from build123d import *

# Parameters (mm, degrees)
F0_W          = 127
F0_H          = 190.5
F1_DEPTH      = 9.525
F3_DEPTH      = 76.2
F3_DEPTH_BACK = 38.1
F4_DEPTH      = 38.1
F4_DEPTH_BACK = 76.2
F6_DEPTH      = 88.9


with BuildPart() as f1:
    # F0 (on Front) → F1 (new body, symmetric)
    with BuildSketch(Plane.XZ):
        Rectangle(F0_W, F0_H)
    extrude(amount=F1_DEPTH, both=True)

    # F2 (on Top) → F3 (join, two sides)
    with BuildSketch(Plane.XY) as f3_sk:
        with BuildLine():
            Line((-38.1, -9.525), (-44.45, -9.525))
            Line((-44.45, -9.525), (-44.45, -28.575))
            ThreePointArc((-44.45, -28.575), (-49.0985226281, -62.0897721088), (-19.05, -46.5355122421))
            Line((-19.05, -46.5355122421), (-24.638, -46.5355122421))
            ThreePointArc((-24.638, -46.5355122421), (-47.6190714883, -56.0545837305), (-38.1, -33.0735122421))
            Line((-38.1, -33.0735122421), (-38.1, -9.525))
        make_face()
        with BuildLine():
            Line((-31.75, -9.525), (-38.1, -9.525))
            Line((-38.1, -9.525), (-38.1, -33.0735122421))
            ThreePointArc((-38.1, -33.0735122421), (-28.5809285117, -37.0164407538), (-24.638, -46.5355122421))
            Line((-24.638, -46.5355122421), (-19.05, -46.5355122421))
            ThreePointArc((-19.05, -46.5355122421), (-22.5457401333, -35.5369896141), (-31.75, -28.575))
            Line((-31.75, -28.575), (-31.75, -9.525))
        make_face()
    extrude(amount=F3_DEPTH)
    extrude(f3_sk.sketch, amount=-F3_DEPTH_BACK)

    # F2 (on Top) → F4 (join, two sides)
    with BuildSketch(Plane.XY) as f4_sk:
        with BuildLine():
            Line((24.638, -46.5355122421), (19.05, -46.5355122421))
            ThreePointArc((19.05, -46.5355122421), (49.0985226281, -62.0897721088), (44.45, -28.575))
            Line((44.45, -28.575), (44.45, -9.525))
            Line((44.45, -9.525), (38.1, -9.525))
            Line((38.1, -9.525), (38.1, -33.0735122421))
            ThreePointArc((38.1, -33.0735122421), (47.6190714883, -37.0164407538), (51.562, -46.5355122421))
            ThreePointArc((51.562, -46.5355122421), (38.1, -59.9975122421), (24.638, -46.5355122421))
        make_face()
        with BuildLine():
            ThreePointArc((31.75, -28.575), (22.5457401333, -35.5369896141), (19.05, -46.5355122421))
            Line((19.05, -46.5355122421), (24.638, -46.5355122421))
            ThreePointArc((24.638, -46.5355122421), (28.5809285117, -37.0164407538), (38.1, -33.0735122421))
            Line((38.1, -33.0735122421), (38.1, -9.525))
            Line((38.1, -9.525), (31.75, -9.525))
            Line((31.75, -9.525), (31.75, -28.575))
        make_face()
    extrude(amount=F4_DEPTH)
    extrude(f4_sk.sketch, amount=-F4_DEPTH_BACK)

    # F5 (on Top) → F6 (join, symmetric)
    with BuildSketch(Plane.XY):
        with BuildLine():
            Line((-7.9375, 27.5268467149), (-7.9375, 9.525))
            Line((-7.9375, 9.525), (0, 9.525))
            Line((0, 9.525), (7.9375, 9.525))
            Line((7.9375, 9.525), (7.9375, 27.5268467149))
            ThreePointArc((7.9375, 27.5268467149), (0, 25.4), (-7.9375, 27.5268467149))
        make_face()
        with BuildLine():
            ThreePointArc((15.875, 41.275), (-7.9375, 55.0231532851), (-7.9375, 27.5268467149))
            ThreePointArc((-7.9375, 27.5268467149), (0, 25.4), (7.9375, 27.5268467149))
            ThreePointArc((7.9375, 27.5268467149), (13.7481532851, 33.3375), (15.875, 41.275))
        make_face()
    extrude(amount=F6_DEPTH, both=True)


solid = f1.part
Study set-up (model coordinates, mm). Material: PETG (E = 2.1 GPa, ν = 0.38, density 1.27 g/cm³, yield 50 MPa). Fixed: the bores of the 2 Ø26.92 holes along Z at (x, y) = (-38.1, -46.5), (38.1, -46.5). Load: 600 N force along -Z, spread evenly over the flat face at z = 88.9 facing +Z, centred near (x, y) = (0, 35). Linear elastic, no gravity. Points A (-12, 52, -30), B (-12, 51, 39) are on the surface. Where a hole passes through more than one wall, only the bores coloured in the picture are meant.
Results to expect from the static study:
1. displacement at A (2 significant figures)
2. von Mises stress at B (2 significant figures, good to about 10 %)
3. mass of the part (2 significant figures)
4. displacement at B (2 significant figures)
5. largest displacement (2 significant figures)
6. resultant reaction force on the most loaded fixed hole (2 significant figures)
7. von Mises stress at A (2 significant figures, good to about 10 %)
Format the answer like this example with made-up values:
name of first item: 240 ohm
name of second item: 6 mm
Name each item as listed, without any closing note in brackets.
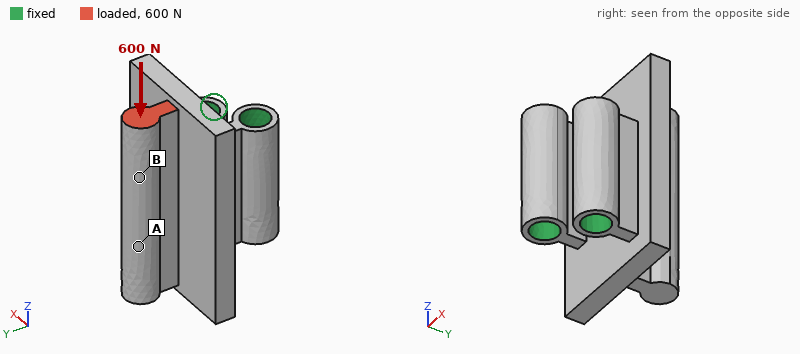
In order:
displacement at A: 45 µm
von Mises stress at B: 0.61 MPa
mass of the part: 1.1 kg
displacement at B: 58 µm
largest displacement: 92 µm
resultant reaction force on the most loaded fixed hole: 310 N
von Mises stress at A: 0.14 MPa
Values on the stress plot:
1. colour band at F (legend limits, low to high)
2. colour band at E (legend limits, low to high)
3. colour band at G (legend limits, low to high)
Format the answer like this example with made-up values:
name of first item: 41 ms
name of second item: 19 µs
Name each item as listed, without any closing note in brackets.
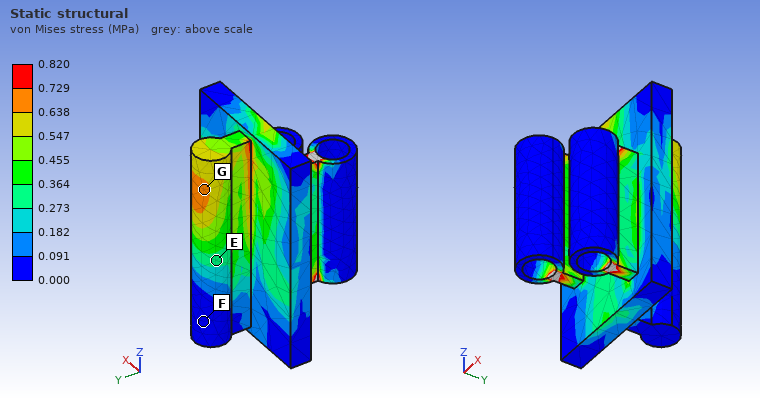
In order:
colour band at F: 0.000 to 0.091 MPa
colour band at E: 0.273 to 0.364 MPa
colour band at G: 0.638 to 0.729 MPa
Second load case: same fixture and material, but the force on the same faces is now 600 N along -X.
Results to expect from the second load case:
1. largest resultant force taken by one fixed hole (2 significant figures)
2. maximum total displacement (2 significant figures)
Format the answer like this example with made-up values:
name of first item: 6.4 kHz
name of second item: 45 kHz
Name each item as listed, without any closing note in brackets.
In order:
largest resultant force taken by one fixed hole: 710 N
maximum total displacement: 0.44 mm
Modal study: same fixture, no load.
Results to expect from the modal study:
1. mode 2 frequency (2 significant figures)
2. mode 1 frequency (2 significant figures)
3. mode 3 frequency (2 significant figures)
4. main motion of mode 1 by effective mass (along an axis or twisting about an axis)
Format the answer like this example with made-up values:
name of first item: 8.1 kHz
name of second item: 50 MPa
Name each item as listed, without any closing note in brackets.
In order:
mode 2 frequency: 880 Hz
mode 1 frequency: 660 Hz
mode 3 frequency: 900 Hz
main motion of mode 1 by effective mass: along X
